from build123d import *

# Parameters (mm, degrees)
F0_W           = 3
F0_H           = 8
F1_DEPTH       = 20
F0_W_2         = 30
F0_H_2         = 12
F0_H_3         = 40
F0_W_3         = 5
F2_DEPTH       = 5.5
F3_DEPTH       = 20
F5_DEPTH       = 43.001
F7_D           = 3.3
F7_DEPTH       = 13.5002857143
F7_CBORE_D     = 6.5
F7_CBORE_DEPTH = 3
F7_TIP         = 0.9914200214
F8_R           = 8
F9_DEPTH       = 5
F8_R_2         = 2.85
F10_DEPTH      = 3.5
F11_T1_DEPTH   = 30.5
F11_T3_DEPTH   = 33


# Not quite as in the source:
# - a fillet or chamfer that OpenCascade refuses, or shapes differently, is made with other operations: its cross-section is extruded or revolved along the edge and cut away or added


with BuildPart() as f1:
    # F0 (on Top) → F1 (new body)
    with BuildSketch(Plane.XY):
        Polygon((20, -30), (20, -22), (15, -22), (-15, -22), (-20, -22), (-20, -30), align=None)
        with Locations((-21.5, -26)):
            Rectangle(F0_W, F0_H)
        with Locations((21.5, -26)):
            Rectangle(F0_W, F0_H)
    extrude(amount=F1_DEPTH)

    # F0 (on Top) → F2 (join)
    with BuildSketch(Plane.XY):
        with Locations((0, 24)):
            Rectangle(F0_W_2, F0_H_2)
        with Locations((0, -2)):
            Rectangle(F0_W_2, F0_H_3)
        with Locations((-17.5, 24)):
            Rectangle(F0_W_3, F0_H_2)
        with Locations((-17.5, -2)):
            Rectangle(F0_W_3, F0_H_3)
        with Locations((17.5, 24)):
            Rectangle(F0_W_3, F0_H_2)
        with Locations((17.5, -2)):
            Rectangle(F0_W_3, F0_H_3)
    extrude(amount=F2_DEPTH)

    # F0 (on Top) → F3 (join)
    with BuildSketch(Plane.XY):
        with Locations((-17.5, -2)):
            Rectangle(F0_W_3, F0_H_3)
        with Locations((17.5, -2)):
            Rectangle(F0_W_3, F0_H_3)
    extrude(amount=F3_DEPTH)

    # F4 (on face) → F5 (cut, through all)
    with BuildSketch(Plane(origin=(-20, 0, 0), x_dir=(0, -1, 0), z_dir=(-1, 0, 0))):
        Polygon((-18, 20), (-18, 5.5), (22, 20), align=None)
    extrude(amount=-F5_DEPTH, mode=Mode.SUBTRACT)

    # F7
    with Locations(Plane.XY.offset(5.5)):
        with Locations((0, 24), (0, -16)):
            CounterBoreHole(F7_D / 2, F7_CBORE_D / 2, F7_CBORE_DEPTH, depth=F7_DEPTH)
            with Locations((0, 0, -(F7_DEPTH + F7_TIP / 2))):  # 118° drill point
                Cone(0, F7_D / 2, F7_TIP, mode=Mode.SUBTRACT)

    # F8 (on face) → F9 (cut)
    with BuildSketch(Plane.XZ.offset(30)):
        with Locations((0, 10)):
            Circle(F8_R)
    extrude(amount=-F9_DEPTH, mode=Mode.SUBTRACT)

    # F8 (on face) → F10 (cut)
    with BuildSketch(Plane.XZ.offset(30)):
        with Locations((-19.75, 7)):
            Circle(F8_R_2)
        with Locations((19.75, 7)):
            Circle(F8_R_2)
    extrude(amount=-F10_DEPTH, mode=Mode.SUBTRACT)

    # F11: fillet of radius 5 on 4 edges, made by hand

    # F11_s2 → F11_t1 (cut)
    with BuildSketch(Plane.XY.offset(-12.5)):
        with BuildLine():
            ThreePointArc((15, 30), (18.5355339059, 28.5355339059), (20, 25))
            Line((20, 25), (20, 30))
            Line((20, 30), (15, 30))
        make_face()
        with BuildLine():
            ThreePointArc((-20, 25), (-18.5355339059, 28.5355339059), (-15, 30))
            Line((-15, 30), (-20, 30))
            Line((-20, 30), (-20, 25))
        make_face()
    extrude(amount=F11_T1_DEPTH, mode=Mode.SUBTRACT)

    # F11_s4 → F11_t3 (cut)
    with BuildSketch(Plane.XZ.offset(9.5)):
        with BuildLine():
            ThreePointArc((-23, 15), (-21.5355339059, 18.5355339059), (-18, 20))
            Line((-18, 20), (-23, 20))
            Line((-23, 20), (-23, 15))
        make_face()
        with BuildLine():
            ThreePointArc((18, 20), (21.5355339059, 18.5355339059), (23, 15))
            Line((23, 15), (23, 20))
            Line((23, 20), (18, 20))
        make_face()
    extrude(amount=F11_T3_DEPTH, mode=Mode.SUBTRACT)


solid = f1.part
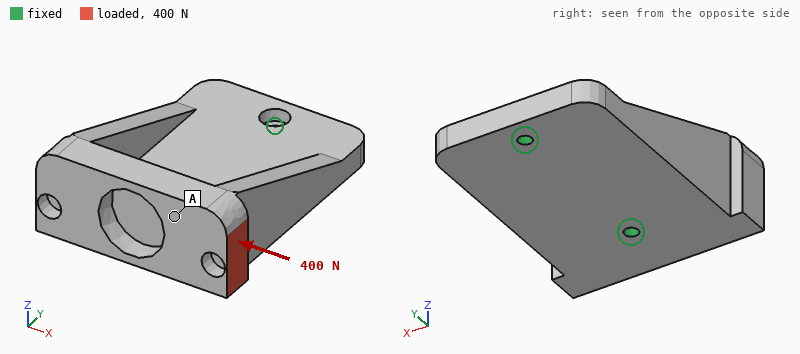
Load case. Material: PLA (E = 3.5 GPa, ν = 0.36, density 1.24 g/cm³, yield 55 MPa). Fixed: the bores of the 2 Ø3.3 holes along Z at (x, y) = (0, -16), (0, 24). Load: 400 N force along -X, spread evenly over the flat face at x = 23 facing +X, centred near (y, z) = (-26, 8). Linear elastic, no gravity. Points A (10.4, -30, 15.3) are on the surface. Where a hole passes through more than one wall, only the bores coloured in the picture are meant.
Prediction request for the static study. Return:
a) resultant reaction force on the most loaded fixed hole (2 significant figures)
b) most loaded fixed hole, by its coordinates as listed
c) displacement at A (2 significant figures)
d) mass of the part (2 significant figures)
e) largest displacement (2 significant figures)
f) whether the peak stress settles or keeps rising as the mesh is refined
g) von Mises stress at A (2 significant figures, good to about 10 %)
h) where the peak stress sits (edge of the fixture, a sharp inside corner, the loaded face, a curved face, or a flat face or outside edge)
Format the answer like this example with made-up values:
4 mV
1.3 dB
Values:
490 N
(0, -16)
0.52 mm
25 g
0.79 mm
keeps rising
5.4 MPa
edge of the fixture
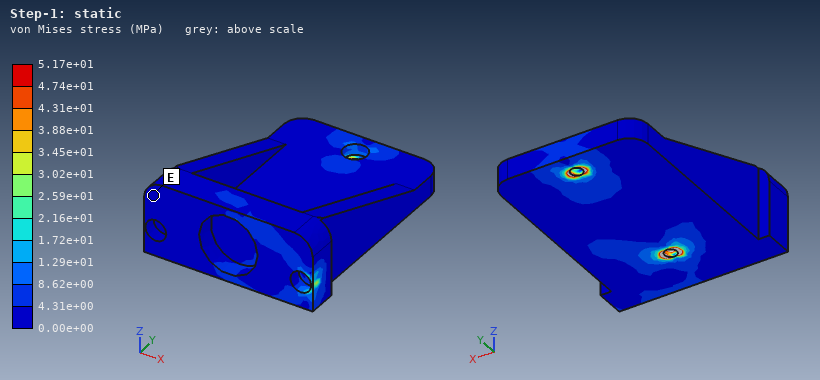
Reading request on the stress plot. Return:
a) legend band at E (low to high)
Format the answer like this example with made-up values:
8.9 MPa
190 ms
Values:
0.00e+00 to 4.31e+00 MPa
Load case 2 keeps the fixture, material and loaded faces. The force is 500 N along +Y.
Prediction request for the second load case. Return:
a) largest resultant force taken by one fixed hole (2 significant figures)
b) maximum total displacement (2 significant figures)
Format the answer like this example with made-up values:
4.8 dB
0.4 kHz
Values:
400 N
0.26 mm
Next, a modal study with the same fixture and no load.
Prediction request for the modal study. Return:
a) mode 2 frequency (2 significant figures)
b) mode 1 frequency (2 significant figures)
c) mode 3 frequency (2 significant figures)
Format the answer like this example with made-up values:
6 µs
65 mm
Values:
2100 Hz
700 Hz
2300 Hz
